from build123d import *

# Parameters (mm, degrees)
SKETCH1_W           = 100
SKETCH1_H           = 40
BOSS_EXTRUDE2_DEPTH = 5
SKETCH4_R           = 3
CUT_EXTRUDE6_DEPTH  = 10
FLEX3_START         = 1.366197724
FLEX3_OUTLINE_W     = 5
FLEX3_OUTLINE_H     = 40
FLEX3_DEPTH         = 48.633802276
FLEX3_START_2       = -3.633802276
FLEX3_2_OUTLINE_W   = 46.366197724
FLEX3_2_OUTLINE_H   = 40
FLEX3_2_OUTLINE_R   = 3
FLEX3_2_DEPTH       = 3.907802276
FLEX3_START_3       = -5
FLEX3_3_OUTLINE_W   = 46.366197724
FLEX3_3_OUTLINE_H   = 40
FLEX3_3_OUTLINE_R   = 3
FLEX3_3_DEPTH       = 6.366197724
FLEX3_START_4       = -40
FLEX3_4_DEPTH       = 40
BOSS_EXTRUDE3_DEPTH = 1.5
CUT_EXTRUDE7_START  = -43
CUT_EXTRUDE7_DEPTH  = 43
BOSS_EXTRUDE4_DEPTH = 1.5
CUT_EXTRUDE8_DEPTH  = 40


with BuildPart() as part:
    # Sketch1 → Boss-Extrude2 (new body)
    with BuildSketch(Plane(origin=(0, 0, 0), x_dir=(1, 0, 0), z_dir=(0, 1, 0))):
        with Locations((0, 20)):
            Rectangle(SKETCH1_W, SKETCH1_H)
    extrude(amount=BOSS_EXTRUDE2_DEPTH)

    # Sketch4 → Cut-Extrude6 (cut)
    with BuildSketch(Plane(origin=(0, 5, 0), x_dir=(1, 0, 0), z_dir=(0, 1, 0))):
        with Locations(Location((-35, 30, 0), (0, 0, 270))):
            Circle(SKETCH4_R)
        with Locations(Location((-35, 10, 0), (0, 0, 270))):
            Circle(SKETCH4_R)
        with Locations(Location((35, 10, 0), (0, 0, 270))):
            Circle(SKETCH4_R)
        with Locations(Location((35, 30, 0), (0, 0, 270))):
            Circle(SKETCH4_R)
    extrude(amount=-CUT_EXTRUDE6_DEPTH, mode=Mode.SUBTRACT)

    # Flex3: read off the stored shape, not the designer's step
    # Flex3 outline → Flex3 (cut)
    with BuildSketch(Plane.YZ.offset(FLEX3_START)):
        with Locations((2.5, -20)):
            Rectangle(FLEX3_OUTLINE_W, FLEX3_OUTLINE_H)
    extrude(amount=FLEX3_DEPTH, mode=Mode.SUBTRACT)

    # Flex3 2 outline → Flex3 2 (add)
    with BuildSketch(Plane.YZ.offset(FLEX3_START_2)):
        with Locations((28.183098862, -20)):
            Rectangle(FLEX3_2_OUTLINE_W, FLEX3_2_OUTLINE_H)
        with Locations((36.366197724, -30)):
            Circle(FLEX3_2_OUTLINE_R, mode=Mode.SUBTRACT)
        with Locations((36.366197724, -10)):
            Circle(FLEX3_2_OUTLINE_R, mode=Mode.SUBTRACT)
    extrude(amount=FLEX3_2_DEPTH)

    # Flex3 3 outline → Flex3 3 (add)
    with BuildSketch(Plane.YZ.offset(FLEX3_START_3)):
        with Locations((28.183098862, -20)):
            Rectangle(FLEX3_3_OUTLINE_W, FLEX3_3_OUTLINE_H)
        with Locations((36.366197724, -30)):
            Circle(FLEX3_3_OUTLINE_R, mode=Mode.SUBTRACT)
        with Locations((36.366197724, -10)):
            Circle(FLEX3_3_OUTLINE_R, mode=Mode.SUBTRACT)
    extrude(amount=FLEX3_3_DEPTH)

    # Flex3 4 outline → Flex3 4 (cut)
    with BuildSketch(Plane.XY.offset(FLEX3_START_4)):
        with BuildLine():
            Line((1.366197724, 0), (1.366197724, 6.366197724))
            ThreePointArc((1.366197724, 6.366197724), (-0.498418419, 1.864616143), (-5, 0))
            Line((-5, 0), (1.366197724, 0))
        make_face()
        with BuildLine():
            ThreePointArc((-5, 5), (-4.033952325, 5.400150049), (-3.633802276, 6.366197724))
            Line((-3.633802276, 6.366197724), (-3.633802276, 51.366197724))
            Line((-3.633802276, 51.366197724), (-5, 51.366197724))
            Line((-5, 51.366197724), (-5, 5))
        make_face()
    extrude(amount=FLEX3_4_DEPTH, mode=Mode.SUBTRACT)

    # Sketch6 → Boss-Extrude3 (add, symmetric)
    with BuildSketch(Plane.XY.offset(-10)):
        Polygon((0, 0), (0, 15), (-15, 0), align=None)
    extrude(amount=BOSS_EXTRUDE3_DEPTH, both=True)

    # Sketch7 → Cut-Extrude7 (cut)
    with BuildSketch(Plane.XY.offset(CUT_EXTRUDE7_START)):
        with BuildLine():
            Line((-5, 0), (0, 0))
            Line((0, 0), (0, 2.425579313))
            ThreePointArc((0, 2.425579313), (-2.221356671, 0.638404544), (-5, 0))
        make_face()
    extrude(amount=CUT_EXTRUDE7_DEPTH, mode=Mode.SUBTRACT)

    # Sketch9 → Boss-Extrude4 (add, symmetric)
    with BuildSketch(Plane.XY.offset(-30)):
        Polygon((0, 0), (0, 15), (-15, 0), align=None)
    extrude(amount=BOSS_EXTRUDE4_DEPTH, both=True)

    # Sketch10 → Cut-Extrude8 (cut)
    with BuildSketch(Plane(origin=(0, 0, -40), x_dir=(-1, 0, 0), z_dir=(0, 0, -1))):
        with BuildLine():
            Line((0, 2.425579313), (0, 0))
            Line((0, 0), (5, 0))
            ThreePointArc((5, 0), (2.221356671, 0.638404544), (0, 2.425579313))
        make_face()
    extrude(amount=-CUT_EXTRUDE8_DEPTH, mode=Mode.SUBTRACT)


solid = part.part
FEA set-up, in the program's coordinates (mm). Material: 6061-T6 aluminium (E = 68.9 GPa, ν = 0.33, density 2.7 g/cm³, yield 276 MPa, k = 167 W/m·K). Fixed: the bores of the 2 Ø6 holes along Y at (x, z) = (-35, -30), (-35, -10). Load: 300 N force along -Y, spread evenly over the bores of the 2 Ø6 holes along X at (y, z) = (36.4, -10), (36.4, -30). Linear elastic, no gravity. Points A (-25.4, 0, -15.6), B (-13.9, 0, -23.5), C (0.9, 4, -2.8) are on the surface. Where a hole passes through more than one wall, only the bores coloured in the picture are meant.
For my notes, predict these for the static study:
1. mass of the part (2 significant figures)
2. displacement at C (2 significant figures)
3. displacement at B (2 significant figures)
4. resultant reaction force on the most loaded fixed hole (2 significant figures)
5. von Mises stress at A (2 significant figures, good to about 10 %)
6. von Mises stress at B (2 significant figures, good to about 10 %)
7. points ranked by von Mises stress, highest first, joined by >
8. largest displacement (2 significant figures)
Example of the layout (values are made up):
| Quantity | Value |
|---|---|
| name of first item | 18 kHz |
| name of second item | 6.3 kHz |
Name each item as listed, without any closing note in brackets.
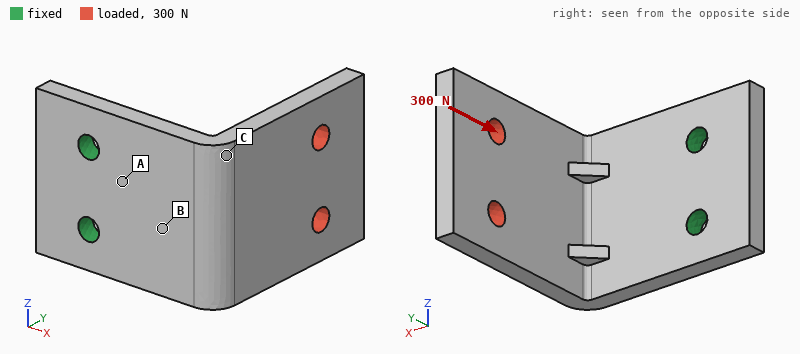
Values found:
| Quantity | Value |
|---|---|
| mass of the part | 51 g |
| displacement at C | 0.13 mm |
| displacement at B | 0.055 mm |
| resultant reaction force on the most loaded fixed hole | 150 N |
| von Mises stress at A | 39 MPa |
| von Mises stress at B | 20 MPa |
| points ranked by von Mises stress, highest first, joined by > | A > B > C |
| largest displacement | 0.29 mm |
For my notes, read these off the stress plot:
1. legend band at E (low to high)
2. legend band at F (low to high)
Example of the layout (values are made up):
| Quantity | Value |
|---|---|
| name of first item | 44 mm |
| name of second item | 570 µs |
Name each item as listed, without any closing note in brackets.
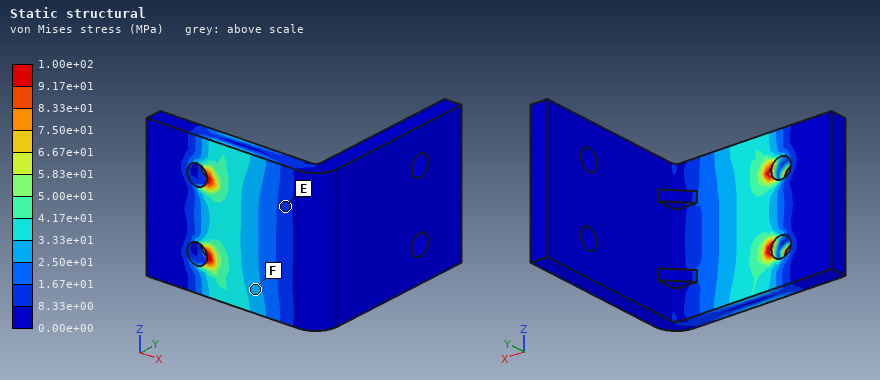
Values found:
| Quantity | Value |
|---|---|
| legend band at E | 8.33e+00 to 1.67e+01 MPa |
| legend band at F | 2.50e+01 to 3.33e+01 MPa |
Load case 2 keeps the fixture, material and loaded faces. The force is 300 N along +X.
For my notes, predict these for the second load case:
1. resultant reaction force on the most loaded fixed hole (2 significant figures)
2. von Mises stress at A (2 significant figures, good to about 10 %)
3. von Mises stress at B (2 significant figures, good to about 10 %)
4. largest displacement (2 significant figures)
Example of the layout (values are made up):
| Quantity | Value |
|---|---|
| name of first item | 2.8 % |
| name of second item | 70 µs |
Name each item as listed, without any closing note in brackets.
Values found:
| Quantity | Value |
|---|---|
| resultant reaction force on the most loaded fixed hole | 160 N |
| von Mises stress at A | 52 MPa |
| von Mises stress at B | 52 MPa |
| largest displacement | 0.68 mm |
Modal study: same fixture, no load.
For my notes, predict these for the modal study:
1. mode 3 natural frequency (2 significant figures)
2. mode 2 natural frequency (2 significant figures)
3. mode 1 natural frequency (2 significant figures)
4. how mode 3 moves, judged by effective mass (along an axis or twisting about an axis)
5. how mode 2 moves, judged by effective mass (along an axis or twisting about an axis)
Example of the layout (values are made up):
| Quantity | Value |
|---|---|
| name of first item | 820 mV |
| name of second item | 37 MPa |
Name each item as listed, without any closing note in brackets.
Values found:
| Quantity | Value |
|---|---|
| mode 3 natural frequency | 2600 Hz |
| mode 2 natural frequency | 1500 Hz |
| mode 1 natural frequency | 870 Hz |
| how mode 3 moves, judged by effective mass | along Y |
| how mode 2 moves, judged by effective mass | along Z |
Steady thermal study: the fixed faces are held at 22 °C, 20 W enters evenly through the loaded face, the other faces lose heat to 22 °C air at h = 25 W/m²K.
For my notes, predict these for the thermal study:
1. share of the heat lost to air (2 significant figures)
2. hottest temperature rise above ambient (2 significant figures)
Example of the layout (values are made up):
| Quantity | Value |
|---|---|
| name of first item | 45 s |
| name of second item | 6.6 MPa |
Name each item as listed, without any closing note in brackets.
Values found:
| Quantity | Value |
|---|---|
| share of the heat lost to air | 18 % |
| hottest temperature rise above ambient | 35 K |
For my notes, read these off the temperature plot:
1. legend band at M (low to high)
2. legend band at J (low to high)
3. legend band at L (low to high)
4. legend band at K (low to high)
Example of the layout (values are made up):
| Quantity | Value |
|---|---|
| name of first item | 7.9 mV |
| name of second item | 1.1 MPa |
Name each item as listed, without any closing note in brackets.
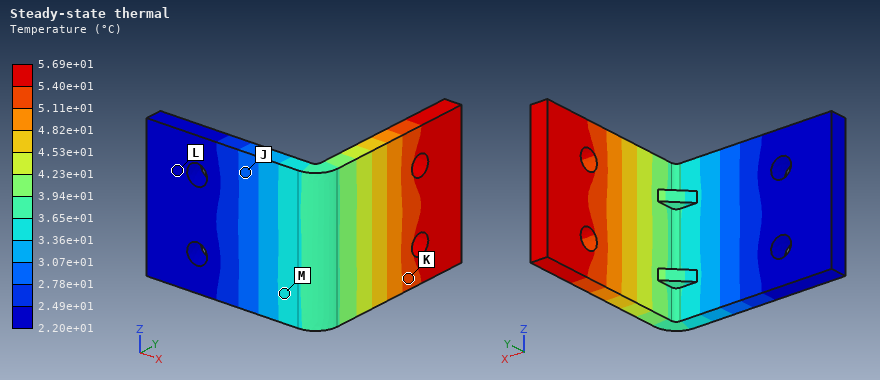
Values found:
| Quantity | Value |
|---|---|
| legend band at M | 3.36e+01 to 3.65e+01 °C |
| legend band at J | 2.78e+01 to 3.07e+01 °C |
| legend band at L | 2.20e+01 to 2.49e+01 °C |
| legend band at K | 5.11e+01 to 5.40e+01 °C |
